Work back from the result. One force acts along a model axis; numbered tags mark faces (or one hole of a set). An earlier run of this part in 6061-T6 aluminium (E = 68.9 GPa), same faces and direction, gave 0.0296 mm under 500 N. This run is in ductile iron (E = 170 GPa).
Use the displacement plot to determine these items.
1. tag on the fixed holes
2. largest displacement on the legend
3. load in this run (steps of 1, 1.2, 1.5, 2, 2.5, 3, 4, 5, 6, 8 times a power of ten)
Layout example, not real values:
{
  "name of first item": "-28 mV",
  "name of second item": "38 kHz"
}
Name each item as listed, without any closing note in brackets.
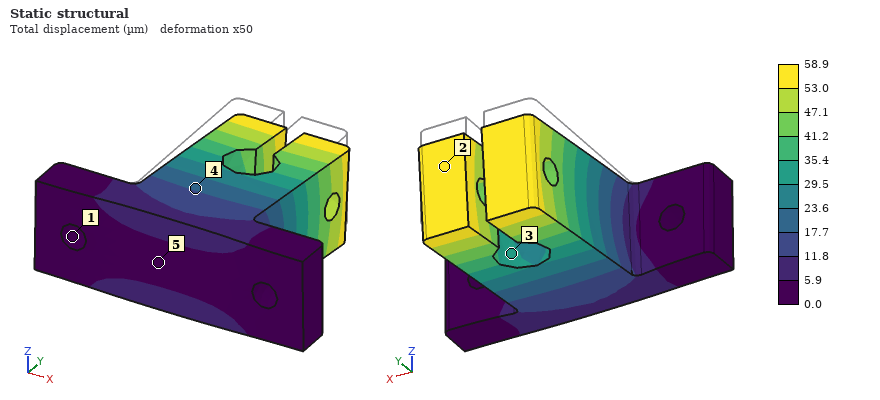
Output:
{
  "tag on the fixed holes": "1",
  "largest displacement on the legend": "58.9 µm",
  "load in this run": "2.5 kN"
}
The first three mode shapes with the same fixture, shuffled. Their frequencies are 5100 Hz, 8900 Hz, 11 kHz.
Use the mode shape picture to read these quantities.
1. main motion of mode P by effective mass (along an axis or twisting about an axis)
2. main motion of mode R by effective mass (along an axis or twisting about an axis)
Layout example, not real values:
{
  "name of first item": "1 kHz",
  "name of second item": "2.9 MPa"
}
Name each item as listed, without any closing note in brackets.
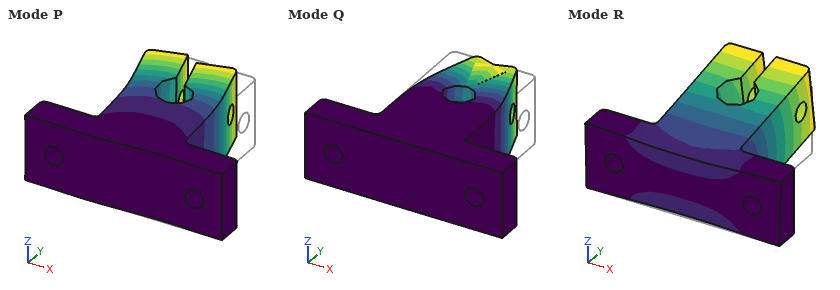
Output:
{
  "main motion of mode P by effective mass": "along X",
  "main motion of mode R by effective mass": "along Z"
}
